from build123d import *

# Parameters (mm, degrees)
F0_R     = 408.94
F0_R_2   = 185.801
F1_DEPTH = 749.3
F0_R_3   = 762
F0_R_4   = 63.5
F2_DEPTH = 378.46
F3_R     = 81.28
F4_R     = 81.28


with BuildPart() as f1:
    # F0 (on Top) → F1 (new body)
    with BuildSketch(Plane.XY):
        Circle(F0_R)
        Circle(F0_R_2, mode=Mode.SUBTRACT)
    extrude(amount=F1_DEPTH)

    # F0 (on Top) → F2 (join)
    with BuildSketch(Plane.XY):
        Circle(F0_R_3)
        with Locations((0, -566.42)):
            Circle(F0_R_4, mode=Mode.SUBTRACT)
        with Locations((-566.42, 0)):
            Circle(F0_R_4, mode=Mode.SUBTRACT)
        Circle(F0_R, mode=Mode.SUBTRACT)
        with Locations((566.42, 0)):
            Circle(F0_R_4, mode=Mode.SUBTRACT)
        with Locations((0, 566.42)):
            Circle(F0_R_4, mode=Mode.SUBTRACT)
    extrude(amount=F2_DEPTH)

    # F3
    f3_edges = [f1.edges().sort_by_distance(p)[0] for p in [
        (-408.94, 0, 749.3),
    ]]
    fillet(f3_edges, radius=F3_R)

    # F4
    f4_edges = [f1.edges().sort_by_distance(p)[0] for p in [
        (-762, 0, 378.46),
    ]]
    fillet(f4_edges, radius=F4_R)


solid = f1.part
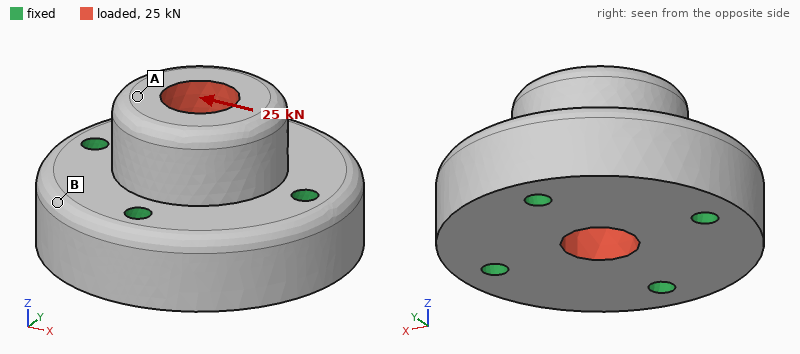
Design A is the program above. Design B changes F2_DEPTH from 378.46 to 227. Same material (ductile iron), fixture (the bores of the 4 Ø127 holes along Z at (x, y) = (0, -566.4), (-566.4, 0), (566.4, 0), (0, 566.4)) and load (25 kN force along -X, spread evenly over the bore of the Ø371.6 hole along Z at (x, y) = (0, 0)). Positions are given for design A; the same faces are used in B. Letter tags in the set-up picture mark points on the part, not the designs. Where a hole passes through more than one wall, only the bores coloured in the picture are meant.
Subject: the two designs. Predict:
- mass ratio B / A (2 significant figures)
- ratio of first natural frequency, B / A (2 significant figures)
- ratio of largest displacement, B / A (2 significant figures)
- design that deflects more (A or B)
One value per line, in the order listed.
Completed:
0.76
0.66
2.2
B
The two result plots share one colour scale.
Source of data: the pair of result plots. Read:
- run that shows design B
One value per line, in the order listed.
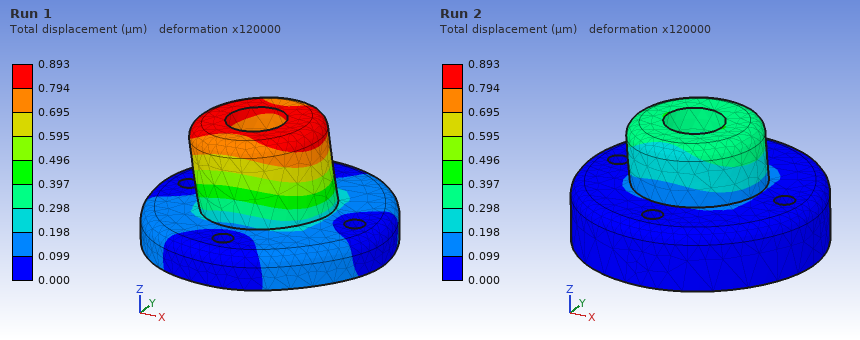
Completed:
Run 1
